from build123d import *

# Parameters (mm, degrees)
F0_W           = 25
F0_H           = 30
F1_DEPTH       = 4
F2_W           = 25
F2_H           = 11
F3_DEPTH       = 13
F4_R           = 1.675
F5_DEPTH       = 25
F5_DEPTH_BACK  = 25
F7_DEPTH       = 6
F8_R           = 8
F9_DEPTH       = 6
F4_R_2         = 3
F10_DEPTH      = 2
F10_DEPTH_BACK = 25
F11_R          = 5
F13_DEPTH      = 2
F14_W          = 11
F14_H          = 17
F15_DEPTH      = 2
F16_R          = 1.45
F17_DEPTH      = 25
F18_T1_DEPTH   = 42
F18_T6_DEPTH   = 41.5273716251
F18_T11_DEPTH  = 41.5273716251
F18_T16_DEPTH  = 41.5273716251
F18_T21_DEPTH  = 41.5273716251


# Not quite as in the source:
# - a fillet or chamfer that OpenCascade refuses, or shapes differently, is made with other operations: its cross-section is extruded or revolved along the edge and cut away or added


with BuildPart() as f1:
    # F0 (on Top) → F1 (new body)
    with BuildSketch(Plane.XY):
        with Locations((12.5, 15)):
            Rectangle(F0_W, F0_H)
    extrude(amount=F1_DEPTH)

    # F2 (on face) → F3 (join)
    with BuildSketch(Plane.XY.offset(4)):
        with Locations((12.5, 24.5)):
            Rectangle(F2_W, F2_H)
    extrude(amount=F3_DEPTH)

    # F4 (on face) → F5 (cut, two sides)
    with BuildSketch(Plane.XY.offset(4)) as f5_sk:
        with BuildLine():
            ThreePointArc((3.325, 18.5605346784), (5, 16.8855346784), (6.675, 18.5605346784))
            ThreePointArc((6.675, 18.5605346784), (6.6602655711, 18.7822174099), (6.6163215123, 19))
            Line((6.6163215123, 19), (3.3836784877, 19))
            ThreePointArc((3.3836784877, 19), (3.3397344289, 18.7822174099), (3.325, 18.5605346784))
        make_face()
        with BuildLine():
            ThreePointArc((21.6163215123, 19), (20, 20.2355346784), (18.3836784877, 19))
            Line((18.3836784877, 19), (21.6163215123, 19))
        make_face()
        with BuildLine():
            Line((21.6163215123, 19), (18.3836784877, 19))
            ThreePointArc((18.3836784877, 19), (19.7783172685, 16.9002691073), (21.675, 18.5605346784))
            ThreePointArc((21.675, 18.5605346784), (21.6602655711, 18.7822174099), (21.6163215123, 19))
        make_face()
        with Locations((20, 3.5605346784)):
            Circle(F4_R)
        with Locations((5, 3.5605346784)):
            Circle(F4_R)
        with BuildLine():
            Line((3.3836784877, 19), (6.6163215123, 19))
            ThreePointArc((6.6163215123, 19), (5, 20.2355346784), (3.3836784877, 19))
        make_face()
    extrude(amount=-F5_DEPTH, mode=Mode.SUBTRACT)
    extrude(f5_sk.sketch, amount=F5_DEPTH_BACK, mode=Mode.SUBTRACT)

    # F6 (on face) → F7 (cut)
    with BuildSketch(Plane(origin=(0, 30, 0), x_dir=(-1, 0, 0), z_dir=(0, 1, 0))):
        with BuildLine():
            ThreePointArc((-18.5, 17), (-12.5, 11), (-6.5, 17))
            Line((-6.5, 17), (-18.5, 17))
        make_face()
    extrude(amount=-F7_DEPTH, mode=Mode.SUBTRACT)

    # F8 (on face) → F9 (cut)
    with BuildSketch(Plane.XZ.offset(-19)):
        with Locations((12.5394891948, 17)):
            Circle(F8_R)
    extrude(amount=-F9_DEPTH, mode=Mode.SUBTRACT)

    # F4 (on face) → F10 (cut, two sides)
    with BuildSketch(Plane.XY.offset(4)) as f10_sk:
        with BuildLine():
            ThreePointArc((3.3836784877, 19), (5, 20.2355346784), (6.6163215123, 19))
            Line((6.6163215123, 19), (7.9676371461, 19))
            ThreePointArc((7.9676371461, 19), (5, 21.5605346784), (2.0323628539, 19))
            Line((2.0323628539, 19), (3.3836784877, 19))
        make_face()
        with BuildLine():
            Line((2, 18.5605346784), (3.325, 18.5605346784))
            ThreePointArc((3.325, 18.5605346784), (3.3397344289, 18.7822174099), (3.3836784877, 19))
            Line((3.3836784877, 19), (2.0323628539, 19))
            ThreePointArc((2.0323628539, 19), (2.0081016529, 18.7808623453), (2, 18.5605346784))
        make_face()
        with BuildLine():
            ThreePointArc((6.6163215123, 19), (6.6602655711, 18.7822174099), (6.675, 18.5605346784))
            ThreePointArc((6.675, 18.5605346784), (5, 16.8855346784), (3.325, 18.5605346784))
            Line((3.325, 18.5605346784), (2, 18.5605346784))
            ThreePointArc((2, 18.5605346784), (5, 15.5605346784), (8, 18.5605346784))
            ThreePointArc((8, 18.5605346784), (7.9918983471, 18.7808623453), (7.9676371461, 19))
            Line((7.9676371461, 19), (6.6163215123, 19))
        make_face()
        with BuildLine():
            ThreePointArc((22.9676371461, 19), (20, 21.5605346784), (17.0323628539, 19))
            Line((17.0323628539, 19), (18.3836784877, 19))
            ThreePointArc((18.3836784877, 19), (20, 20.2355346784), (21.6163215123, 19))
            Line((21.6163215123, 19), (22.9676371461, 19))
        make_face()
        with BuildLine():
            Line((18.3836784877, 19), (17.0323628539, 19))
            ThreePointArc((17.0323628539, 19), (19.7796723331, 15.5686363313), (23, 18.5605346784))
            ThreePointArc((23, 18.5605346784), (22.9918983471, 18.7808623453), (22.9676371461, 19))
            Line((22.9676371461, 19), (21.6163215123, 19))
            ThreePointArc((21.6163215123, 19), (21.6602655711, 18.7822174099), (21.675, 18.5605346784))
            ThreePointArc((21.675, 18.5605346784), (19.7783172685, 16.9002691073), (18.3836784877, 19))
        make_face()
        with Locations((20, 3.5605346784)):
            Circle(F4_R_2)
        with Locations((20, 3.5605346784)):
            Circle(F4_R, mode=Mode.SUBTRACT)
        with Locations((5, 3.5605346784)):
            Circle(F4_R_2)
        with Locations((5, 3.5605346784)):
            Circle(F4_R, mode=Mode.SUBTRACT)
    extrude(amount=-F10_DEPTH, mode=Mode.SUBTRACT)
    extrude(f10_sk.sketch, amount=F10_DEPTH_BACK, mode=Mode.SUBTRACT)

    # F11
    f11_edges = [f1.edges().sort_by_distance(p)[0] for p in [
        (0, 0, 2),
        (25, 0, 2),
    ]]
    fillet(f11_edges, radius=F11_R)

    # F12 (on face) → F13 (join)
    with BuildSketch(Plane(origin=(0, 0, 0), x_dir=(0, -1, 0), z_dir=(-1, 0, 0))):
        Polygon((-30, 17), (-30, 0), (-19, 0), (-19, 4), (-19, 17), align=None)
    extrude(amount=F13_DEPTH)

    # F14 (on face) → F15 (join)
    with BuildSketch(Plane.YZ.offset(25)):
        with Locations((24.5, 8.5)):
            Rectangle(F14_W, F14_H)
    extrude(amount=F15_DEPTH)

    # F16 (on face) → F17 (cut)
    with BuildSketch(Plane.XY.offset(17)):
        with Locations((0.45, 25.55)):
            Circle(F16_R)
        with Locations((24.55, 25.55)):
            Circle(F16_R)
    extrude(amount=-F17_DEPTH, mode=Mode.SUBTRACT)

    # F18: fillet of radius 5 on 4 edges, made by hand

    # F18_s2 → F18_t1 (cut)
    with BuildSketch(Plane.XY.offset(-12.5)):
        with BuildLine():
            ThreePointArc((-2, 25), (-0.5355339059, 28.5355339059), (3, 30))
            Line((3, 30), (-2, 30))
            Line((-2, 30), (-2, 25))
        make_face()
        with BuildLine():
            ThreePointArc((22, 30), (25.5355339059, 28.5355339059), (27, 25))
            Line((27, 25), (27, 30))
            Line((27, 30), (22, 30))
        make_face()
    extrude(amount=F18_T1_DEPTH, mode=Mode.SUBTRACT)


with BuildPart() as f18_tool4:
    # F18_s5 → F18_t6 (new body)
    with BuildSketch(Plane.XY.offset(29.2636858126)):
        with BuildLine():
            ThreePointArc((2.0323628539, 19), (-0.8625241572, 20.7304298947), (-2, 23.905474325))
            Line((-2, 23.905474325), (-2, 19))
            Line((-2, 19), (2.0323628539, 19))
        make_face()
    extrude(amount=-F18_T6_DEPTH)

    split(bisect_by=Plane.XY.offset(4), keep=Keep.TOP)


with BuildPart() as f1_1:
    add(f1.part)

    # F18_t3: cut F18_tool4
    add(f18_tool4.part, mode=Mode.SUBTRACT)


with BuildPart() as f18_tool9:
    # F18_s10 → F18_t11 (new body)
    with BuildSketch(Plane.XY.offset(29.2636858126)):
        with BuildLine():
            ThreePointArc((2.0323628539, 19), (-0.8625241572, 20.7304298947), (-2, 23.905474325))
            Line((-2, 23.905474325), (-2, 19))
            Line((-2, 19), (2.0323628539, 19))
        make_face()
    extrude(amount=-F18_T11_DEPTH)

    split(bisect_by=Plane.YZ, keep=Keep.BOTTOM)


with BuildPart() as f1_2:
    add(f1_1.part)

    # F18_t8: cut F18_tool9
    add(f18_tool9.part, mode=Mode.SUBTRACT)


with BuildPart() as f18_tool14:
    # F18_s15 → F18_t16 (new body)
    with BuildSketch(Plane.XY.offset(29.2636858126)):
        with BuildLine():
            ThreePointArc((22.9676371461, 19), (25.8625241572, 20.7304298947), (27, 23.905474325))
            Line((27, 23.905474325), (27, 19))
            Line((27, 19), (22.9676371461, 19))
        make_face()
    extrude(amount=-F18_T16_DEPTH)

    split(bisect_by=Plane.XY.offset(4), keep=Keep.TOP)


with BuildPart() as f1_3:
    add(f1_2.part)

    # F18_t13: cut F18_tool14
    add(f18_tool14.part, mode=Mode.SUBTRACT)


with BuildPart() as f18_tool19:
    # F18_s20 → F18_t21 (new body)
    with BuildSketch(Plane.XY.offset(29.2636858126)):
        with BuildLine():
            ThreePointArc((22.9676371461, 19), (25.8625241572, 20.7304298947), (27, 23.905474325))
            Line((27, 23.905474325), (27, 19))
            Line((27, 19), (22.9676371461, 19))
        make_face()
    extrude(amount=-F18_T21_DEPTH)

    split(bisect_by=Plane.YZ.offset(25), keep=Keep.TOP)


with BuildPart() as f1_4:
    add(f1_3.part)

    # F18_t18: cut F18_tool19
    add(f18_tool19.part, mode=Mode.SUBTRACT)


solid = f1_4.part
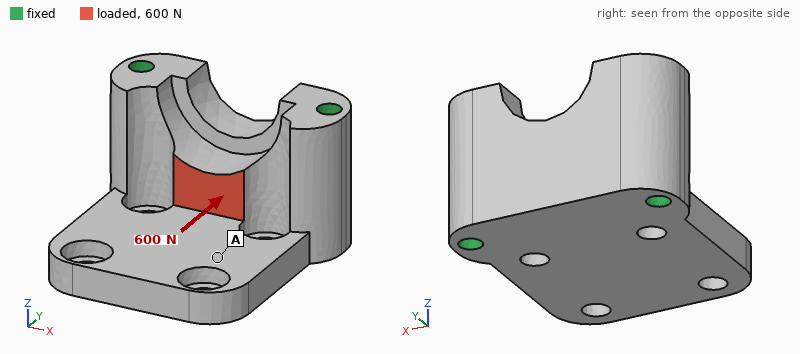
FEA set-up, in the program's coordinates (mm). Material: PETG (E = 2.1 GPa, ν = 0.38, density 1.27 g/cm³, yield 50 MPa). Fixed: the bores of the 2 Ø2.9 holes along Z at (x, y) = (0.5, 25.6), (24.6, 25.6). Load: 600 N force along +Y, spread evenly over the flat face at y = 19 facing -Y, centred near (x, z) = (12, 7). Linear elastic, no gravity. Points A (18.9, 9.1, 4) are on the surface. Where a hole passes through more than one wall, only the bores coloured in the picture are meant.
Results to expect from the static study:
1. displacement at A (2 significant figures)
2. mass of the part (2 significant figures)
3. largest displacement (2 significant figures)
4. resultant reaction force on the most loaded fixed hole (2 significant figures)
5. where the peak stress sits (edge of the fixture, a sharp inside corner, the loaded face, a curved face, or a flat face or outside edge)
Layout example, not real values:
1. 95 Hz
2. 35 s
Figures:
1. 53 µm
2. 6.7 g
3. 90 µm
4. 310 N
5. a curved face
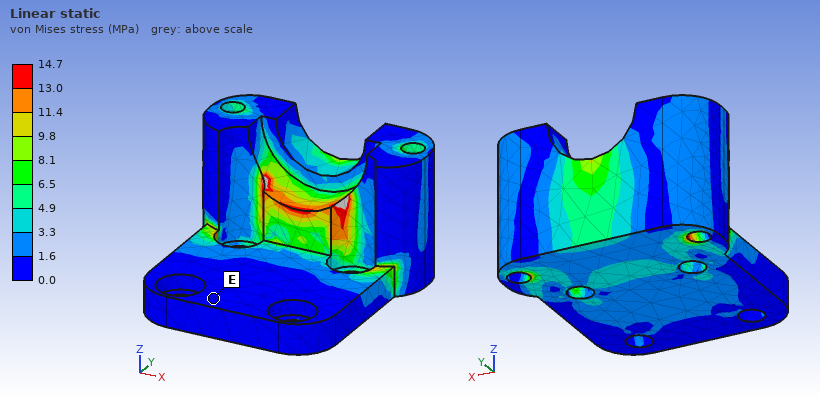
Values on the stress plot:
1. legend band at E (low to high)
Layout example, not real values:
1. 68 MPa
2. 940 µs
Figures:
1. 0.0 to 1.6 MPa
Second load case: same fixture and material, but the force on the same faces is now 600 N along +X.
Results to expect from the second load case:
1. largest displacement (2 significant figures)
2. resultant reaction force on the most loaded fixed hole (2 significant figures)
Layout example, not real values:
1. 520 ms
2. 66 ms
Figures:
1. 85 µm
2. 350 N
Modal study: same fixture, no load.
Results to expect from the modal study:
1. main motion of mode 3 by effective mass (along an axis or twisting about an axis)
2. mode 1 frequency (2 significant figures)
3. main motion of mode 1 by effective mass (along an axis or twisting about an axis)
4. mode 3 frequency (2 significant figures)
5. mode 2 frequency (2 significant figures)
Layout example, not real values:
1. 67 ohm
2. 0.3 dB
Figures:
1. along X
2. 1700 Hz
3. along Z
4. 5700 Hz
5. 3700 Hz
